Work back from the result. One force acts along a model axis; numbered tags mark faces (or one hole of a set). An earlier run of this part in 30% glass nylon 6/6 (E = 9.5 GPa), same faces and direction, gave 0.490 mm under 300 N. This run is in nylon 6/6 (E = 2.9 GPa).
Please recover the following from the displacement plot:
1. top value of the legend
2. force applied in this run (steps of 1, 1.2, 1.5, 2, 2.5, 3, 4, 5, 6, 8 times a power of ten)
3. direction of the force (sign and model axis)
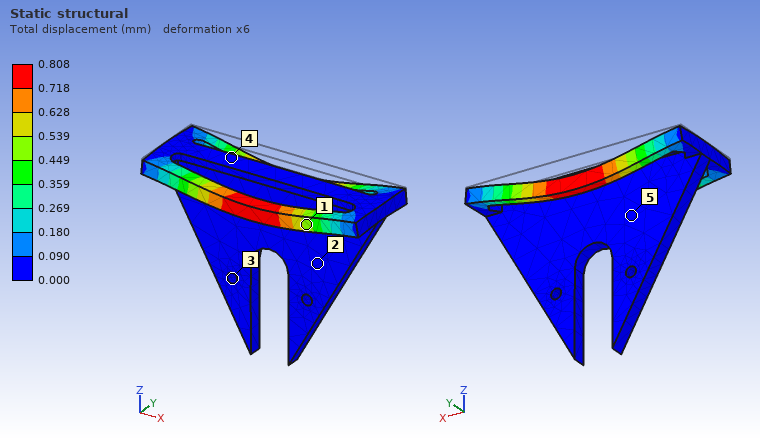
0.808 mm
150 N
-Z
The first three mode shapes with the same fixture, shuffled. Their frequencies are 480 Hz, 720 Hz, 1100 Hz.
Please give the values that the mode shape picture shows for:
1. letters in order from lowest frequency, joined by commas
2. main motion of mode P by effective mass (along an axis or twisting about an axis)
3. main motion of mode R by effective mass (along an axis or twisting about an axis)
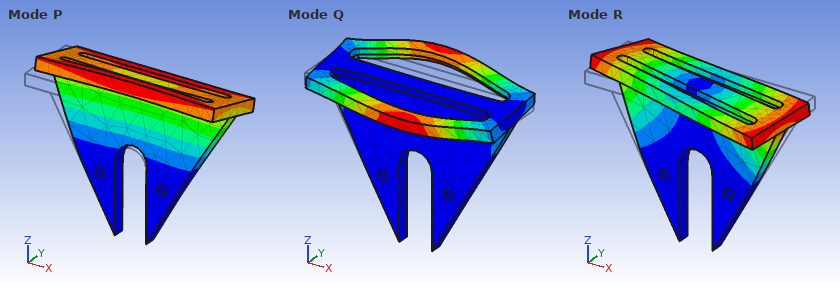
P, R, Q
along Y
twisting about Z
